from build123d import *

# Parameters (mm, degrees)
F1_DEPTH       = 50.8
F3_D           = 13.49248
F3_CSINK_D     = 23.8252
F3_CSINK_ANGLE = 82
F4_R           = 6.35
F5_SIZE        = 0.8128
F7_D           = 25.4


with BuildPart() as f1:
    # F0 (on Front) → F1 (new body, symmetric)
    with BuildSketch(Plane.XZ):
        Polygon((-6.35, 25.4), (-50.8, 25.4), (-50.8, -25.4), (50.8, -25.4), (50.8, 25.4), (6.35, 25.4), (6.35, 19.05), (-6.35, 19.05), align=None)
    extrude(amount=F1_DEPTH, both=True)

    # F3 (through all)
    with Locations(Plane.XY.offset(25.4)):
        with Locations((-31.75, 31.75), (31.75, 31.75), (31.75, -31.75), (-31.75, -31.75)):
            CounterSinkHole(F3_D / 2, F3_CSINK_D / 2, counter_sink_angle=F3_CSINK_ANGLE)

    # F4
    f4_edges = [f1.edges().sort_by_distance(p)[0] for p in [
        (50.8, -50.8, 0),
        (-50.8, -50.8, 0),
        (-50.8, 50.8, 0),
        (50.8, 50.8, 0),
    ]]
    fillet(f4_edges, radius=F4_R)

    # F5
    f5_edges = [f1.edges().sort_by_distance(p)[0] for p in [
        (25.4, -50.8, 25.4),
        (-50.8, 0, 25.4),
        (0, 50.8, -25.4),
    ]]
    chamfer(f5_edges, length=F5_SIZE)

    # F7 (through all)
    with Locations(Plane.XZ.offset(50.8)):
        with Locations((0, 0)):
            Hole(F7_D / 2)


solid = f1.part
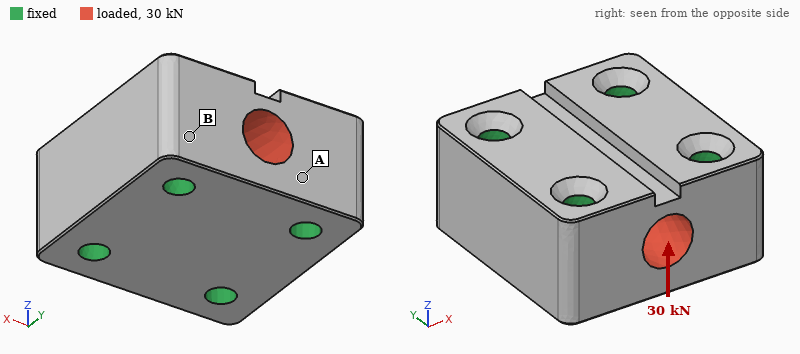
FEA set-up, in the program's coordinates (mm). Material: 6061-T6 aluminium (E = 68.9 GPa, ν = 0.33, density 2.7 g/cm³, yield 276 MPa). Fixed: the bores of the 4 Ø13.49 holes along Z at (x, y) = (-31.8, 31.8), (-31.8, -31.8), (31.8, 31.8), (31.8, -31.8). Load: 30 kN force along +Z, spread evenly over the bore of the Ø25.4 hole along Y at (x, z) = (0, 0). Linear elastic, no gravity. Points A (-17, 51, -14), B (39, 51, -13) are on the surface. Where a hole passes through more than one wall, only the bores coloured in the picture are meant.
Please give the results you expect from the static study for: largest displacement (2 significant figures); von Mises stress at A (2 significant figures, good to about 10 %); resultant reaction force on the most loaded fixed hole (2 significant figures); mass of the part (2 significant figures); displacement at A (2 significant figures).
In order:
7.1 µm
4.8 MPa
7.5 kN
1.2 kg
2.1 µm
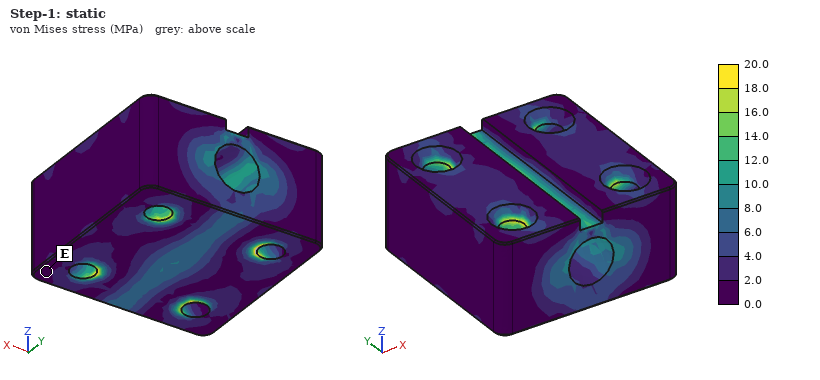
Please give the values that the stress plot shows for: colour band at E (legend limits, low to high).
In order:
0.0 to 2.0 MPa
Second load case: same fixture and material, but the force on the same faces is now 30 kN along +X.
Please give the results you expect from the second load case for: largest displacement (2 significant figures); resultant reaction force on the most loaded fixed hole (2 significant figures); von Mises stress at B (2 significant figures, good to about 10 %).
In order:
2.5 µm
7.6 kN
1.00 MPa
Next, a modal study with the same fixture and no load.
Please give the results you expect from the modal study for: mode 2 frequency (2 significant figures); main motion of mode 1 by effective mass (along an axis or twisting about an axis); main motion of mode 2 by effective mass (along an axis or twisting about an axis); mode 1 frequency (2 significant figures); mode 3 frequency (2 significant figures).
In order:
22 kHz
along Z
along X
20 kHz
23 kHz
